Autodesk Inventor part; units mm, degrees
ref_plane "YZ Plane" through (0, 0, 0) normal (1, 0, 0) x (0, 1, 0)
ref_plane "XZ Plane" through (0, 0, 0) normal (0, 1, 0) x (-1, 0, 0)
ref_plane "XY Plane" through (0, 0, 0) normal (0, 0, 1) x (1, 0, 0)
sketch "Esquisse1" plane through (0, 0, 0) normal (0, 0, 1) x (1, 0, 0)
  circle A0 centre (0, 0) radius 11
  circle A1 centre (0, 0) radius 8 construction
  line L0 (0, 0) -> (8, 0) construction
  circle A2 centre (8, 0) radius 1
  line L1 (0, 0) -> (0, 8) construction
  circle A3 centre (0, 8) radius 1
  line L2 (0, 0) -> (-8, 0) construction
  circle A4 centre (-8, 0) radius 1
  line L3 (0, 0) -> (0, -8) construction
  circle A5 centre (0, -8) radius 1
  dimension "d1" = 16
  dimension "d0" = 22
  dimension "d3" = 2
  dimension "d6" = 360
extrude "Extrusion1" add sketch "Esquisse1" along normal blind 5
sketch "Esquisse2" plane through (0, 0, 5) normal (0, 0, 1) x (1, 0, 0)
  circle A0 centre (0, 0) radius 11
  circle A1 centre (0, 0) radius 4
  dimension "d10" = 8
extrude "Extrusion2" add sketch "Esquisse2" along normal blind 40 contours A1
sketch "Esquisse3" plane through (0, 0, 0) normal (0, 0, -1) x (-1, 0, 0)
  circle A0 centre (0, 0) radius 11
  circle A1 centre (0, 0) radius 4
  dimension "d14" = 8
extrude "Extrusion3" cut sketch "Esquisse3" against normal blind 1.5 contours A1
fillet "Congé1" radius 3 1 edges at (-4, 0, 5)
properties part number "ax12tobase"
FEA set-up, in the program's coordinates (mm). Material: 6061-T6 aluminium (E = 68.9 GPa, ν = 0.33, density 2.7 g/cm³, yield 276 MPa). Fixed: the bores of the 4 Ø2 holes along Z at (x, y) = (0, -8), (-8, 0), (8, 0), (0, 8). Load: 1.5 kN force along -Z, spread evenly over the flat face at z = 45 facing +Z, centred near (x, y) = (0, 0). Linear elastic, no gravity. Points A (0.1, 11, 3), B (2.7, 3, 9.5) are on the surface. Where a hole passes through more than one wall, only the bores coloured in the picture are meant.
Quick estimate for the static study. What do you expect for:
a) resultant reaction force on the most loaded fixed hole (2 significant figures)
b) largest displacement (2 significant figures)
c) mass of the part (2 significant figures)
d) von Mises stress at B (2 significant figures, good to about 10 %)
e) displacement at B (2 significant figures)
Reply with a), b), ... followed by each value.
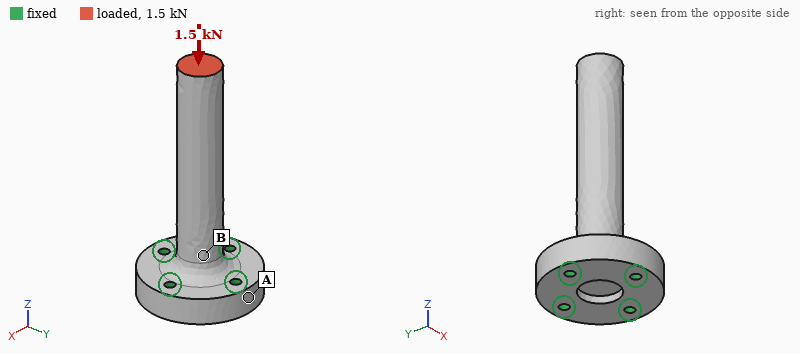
a) 410 N
b) 20 µm
c) 10 g
d) 31 MPa
e) 4.2 µm
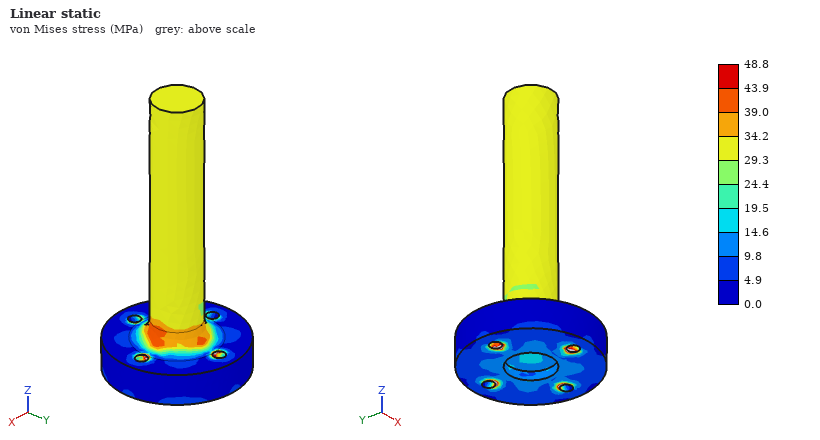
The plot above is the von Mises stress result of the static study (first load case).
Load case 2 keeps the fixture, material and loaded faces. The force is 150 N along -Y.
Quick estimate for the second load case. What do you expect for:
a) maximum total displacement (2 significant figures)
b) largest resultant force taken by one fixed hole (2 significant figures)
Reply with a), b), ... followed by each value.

a) 0.24 mm
b) 410 N
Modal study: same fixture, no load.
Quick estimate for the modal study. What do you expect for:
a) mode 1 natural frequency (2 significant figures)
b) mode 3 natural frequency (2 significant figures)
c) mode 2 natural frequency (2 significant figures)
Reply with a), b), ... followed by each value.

a) 3400 Hz
b) 19 kHz
c) 3400 Hz
